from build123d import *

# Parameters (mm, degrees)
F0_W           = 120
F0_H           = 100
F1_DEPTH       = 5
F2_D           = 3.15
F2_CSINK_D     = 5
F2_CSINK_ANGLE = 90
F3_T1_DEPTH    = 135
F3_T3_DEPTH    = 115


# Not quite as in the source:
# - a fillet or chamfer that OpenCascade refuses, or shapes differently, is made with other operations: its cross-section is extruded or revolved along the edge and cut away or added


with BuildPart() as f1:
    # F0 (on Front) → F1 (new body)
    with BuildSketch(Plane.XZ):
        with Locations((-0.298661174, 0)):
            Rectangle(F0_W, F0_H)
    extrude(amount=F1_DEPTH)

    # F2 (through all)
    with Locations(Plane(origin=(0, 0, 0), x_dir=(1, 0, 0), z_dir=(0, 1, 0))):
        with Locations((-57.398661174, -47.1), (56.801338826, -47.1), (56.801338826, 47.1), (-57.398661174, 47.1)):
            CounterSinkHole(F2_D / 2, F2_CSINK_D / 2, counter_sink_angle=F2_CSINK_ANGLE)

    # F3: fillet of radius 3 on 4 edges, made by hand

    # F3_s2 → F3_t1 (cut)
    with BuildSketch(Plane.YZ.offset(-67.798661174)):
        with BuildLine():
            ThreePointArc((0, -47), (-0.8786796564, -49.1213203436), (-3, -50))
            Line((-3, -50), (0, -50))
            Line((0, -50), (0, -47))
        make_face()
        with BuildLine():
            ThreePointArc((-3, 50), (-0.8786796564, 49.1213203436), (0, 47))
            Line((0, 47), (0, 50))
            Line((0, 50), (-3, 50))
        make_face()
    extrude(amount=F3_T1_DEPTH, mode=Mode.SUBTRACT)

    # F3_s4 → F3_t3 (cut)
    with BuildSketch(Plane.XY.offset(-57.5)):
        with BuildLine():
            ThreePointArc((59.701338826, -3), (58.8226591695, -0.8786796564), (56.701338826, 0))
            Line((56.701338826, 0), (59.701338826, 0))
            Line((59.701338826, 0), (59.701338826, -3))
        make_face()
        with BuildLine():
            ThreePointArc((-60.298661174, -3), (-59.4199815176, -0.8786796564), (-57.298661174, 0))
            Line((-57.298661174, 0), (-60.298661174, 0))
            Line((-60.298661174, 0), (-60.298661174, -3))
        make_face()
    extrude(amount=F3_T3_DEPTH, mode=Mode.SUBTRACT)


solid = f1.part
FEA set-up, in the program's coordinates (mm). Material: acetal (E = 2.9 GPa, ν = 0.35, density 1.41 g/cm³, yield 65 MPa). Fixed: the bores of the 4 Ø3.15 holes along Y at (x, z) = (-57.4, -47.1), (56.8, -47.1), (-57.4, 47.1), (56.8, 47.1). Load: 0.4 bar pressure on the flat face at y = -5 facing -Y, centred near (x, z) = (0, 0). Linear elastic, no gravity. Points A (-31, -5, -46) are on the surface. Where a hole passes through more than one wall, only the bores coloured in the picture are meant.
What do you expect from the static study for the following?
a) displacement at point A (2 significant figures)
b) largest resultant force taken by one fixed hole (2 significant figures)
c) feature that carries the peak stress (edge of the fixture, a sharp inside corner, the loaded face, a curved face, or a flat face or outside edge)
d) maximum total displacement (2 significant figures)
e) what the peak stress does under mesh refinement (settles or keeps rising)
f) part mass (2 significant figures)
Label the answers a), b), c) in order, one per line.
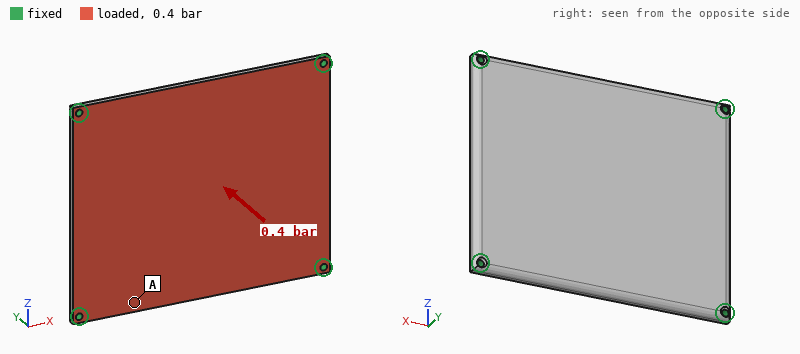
a) 0.79 mm
b) 130 N
c) edge of the fixture
d) 1.7 mm
e) keeps rising
f) 83 g
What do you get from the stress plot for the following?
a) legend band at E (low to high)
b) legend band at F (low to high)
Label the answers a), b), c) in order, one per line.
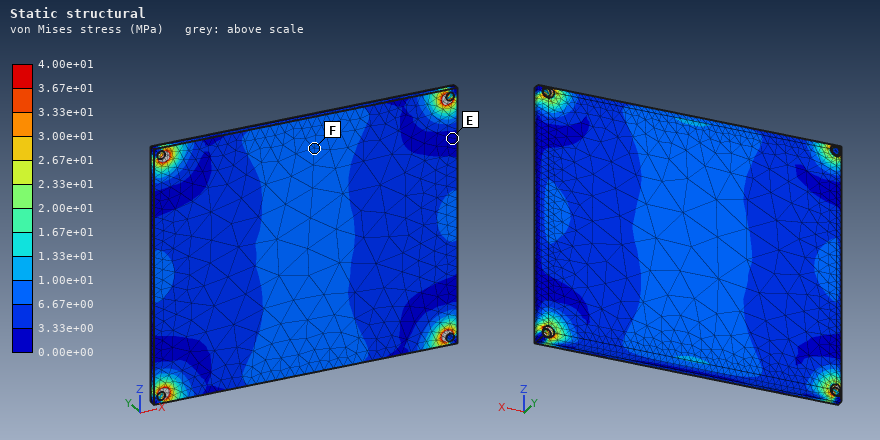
a) 0.00e+00 to 3.33e+00 MPa
b) 6.67e+00 to 1.00e+01 MPa
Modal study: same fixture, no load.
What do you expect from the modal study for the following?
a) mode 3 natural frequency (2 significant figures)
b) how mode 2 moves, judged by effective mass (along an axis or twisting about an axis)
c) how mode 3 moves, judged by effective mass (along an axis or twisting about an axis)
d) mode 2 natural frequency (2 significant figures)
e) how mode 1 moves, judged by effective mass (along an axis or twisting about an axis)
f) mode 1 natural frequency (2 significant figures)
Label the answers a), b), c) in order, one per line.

a) 720 Hz
b) twisting about X
c) twisting about Z
d) 610 Hz
e) along Y
f) 340 Hz
